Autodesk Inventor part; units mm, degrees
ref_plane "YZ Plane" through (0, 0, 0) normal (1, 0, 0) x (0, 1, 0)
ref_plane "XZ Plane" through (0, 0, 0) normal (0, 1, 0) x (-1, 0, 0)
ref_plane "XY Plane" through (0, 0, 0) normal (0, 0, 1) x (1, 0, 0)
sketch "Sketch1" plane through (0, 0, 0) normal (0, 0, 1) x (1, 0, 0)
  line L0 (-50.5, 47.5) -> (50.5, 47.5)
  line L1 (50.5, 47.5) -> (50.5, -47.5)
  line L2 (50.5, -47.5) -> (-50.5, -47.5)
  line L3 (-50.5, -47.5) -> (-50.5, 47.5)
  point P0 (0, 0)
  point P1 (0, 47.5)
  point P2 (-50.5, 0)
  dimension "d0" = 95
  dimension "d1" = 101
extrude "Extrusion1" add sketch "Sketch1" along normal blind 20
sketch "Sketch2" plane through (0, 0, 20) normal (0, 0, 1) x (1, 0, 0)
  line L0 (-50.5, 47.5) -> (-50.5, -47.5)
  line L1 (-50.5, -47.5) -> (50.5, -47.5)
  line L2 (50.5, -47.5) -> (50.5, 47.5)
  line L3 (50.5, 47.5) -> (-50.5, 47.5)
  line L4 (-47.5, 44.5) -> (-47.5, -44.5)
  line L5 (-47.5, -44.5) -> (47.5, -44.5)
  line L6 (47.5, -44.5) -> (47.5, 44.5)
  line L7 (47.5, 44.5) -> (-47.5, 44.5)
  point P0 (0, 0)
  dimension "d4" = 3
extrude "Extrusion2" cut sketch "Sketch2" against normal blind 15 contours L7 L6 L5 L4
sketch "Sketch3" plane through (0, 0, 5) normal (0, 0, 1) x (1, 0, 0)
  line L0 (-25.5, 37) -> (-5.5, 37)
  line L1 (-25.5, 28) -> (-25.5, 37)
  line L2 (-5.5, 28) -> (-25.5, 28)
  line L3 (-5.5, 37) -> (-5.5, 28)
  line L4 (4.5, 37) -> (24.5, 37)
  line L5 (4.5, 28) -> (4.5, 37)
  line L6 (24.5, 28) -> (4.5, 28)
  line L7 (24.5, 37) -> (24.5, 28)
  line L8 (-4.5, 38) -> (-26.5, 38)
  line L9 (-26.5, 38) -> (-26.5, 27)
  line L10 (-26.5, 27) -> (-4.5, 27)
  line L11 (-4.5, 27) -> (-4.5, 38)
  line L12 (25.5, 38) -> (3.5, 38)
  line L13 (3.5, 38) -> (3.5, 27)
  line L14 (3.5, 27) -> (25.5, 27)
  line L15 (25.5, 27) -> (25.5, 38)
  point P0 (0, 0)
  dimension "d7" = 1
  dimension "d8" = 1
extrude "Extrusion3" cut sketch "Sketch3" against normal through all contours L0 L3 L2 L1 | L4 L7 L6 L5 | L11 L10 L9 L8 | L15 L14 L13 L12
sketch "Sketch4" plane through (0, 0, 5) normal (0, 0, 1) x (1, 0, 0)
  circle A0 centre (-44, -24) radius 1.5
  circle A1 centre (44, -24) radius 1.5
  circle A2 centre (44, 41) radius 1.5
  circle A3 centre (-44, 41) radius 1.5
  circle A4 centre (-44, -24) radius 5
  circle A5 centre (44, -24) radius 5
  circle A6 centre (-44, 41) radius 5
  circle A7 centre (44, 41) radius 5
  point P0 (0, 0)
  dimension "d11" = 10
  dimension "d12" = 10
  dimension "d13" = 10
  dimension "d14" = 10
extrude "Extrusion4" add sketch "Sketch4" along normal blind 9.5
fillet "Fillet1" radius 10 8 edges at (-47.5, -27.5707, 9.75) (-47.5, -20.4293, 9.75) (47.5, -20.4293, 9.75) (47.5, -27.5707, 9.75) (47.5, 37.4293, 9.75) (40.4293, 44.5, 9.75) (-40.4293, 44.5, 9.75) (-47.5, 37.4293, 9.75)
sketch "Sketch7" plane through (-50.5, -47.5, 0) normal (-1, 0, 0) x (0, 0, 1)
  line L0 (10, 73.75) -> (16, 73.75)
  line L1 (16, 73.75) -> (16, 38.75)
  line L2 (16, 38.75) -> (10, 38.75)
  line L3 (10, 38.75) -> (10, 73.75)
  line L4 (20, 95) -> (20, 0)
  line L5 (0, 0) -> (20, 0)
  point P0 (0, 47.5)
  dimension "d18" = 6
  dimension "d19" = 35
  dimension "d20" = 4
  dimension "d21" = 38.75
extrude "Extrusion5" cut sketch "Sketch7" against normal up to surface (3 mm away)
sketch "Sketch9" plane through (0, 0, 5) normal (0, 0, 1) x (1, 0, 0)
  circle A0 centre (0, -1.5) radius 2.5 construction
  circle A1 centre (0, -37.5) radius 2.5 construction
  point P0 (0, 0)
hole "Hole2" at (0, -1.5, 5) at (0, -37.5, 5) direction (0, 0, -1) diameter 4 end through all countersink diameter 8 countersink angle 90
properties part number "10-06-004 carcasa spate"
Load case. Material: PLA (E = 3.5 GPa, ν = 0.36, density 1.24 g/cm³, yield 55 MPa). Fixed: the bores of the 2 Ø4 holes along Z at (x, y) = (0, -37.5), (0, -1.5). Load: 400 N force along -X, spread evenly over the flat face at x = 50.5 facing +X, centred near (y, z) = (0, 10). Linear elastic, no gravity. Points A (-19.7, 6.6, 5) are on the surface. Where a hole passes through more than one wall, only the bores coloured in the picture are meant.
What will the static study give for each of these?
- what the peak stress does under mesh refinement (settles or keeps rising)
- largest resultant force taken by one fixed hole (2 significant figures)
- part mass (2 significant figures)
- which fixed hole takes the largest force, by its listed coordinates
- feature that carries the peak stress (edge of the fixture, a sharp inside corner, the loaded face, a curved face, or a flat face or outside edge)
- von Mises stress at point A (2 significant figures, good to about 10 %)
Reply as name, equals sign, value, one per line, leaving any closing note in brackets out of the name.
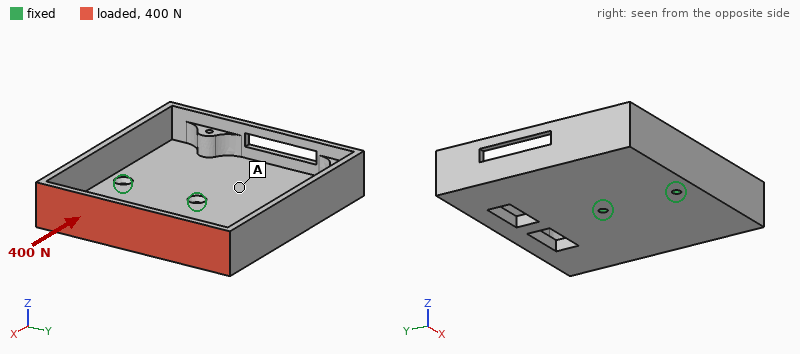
what the peak stress does under mesh refinement = keeps rising
largest resultant force taken by one fixed hole = 410 N
part mass = 81 g
which fixed hole takes the largest force, by its listed coordinates = (0, -1.5)
feature that carries the peak stress = edge of the fixture
von Mises stress at point A = 2.3 MPa
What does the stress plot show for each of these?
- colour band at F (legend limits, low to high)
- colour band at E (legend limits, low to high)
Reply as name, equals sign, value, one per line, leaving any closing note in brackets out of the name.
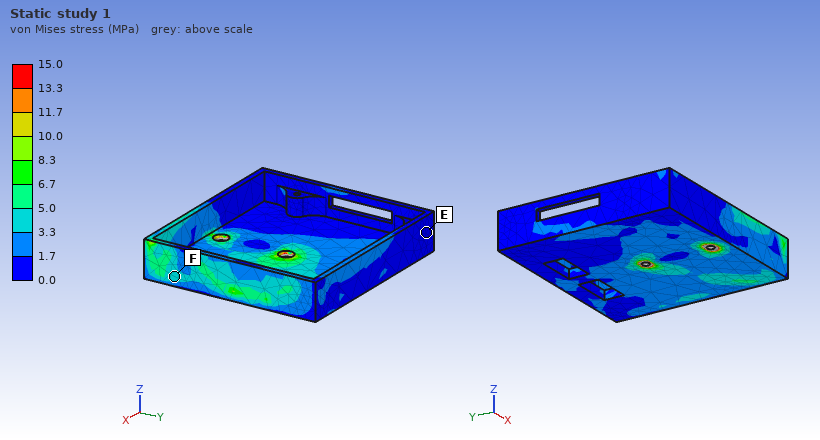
colour band at F = 3.3 to 5.0 MPa
colour band at E = 0.0 to 1.7 MPa
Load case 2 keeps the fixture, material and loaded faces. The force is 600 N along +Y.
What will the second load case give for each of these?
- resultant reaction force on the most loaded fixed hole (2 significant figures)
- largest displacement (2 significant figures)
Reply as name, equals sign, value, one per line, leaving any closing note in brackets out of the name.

resultant reaction force on the most loaded fixed hole = 890 N
largest displacement = 1.7 mm
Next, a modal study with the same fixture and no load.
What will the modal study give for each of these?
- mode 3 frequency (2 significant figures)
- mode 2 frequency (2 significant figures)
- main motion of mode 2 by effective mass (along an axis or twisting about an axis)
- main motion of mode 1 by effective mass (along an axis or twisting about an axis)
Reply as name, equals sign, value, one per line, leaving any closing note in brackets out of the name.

mode 3 frequency = 480 Hz
mode 2 frequency = 340 Hz
main motion of mode 2 by effective mass = along Z
main motion of mode 1 by effective mass = twisting about Y
